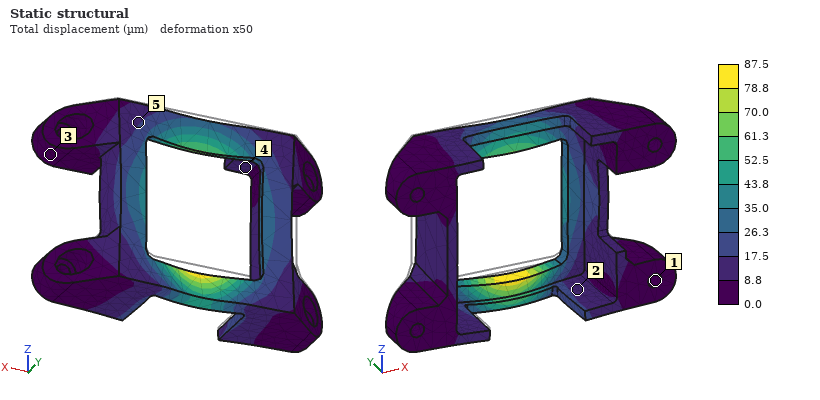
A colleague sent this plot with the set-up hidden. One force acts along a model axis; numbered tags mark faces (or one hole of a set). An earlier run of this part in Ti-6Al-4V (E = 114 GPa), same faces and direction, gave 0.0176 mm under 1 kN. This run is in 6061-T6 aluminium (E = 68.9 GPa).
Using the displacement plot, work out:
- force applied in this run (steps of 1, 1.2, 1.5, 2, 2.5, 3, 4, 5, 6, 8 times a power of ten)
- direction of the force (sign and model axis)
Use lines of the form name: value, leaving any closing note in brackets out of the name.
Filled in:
force applied in this run: 3 kN
direction of the force: -Y
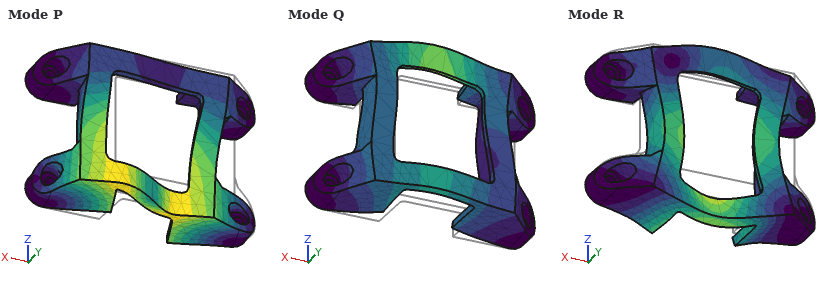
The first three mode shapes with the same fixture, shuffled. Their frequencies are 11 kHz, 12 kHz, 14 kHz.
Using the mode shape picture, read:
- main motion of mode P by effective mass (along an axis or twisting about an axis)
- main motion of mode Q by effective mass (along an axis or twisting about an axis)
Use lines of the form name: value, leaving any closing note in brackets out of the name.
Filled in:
main motion of mode P by effective mass: along X
main motion of mode Q by effective mass: along Z
